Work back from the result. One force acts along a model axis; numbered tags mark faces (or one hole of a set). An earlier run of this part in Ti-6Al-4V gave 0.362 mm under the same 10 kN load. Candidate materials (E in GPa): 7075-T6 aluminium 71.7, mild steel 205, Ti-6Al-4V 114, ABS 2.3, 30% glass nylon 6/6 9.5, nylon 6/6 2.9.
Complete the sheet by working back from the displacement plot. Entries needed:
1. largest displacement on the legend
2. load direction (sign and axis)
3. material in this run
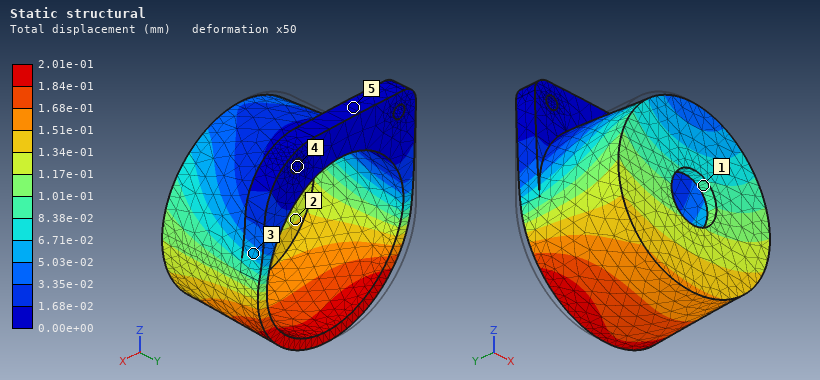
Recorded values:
2.01e-01 mm
+X
mild steel
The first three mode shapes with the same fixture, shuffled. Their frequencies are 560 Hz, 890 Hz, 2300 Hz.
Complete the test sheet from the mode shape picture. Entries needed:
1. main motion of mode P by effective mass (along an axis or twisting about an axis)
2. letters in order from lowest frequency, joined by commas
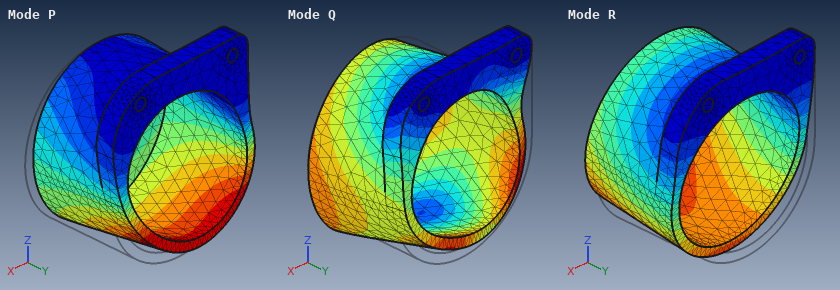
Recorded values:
along X
R, P, Q
